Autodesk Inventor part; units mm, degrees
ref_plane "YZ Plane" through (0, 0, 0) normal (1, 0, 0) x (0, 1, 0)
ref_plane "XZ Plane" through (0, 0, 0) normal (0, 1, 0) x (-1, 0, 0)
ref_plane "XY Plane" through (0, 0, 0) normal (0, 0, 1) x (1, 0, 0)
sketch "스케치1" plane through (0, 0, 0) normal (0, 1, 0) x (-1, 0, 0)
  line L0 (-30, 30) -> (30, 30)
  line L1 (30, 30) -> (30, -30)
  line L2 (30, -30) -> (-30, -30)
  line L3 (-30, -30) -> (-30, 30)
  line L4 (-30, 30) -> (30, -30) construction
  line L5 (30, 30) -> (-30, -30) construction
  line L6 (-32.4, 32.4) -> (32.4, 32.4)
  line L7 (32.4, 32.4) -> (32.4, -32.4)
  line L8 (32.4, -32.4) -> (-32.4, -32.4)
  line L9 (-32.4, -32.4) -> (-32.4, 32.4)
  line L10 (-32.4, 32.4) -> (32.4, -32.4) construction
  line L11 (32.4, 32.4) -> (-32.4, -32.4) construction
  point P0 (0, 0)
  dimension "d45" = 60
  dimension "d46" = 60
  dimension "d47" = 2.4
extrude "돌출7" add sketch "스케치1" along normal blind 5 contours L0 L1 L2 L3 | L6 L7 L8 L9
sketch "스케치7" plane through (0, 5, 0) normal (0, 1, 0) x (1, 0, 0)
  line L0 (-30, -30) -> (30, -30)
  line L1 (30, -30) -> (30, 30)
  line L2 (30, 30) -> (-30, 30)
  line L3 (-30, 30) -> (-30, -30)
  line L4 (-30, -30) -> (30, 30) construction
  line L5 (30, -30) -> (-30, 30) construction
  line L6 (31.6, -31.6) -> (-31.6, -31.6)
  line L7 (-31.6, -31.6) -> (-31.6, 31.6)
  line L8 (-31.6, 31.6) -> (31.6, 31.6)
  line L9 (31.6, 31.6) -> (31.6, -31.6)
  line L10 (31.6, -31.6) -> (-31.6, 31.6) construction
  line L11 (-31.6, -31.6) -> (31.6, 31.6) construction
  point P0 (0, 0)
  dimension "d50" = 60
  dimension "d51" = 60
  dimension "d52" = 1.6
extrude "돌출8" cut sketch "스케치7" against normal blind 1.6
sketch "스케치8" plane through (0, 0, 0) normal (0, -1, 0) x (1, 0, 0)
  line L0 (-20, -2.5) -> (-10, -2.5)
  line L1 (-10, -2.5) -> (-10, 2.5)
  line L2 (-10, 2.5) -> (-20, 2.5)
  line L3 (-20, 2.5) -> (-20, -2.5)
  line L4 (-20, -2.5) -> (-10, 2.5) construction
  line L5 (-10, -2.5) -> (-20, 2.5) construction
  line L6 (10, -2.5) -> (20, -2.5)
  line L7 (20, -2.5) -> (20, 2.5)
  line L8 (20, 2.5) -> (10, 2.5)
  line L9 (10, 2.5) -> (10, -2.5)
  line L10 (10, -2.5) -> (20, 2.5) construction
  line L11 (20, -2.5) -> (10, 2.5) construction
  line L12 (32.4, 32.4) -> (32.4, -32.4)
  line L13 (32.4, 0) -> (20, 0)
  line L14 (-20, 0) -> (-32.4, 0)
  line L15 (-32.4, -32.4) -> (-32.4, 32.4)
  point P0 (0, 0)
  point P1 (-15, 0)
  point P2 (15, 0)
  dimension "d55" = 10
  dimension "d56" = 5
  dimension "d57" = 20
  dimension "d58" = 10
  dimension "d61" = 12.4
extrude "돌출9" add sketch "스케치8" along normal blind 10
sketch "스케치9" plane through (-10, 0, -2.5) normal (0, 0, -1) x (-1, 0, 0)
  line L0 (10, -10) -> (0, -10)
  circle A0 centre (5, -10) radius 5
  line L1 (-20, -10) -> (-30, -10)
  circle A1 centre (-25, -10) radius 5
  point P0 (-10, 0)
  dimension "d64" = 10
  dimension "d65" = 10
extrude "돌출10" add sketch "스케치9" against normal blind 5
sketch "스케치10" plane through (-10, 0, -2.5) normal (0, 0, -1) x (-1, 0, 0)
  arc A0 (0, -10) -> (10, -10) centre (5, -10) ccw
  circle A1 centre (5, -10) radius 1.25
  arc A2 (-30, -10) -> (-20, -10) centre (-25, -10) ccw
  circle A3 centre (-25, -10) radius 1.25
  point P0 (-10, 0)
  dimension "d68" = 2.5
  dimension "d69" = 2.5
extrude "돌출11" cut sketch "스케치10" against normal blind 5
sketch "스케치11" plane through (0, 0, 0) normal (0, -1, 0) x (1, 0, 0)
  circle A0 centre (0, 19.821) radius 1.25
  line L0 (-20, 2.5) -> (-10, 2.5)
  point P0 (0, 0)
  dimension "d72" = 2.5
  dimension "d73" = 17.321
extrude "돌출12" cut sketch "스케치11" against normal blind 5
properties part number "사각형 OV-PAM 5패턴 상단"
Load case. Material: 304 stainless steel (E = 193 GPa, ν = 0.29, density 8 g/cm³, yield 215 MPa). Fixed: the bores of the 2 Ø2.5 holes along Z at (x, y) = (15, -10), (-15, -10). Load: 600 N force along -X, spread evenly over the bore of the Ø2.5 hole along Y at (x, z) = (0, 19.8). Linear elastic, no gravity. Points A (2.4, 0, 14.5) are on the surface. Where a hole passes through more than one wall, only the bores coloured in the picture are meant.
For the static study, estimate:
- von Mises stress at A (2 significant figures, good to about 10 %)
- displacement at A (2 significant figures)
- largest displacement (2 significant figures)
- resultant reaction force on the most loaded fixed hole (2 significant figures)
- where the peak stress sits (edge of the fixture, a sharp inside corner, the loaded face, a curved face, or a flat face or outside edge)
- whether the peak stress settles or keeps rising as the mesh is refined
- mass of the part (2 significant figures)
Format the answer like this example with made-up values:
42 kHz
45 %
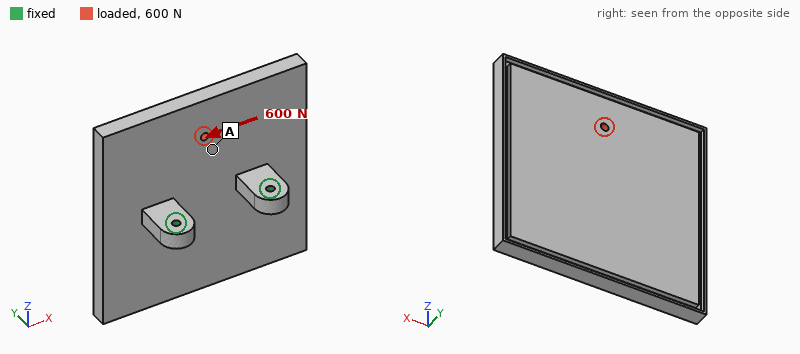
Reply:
7.8 MPa
8.7 µm
18 µm
490 N
edge of the fixture
keeps rising
170 g
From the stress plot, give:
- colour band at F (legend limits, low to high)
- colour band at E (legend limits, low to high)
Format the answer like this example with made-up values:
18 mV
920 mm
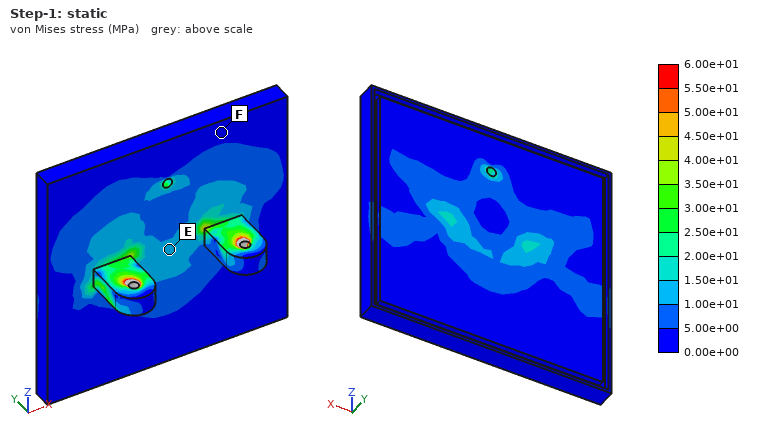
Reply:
0.00e+00 to 5.00e+00 MPa
1.00e+01 to 1.50e+01 MPa
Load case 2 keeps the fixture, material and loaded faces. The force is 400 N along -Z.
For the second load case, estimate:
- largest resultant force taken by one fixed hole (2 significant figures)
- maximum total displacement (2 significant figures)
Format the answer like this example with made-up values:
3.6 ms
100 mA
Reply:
200 N
28 µm
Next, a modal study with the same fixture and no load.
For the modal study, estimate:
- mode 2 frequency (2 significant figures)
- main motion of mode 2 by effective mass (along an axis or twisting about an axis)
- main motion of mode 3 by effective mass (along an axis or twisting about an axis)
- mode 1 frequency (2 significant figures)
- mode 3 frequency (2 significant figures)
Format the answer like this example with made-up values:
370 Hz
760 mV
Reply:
2700 Hz
twisting about Y
along Y
1100 Hz
3900 Hz
